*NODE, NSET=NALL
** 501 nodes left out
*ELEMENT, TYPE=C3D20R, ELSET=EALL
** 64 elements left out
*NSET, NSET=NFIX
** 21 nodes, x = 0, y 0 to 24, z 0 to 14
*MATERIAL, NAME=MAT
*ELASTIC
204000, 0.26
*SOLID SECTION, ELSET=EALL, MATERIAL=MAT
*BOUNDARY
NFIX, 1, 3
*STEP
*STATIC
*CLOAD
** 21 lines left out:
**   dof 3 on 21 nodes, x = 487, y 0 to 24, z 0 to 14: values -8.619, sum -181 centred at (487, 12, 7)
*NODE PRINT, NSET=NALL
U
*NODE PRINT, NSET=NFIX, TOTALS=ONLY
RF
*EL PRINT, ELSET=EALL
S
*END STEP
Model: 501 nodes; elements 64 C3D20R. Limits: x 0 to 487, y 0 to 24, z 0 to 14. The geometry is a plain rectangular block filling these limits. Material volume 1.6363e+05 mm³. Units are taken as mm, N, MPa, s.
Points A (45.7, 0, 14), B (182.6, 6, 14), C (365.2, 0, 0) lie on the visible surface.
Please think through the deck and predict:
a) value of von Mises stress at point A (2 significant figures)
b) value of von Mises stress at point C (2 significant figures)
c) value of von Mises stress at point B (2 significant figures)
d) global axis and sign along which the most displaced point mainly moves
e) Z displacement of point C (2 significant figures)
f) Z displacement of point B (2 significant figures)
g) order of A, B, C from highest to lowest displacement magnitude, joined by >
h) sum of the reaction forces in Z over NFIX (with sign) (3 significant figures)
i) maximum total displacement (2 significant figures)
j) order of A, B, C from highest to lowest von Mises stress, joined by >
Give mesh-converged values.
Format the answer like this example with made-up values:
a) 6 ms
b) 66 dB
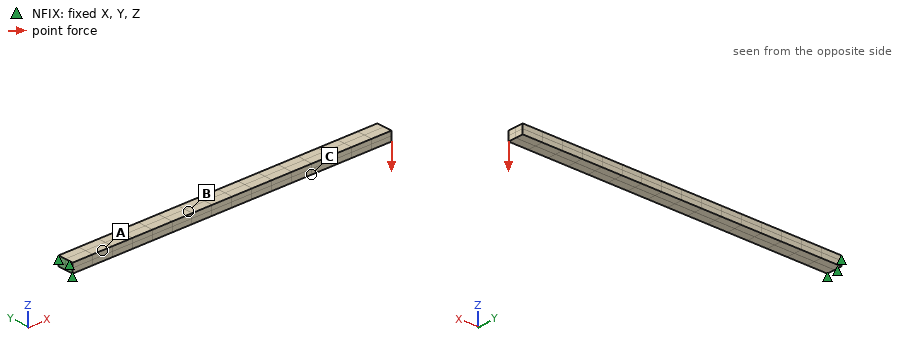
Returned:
a) 100 MPa
b) 28 MPa
c) 70 MPa
d) -Z
e) -3.9 mm
f) -1.1 mm
g) C > B > A
h) 181 N
i) 6.2 mm
j) A > B > C
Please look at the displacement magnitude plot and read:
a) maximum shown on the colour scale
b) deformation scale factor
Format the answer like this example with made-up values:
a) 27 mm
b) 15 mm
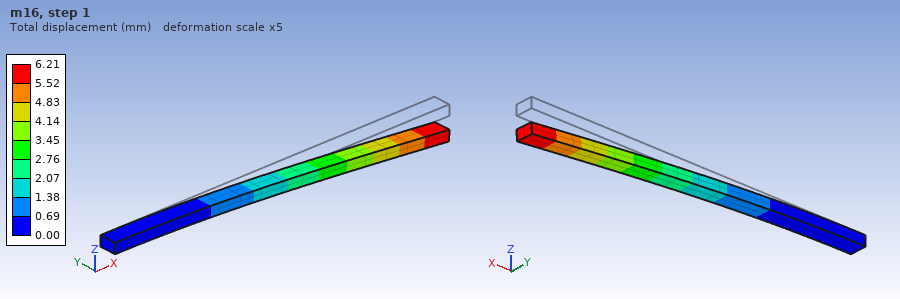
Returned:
a) 6.21 mm
b) 5
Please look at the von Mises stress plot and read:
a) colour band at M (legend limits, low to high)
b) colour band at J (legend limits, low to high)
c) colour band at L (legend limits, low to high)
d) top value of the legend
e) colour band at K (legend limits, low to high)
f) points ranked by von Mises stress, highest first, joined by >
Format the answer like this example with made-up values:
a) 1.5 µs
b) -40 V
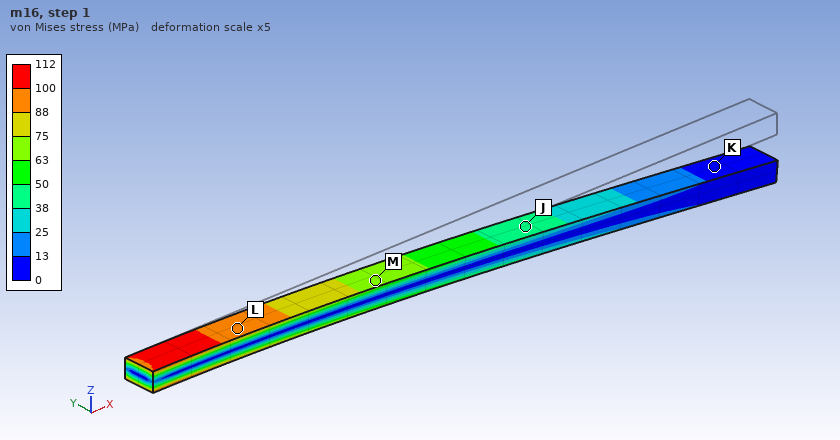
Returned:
a) 63 to 75 MPa
b) 38 to 50 MPa
c) 88 to 100 MPa
d) 112 MPa
e) 0 to 13 MPa
f) L > M > J > K
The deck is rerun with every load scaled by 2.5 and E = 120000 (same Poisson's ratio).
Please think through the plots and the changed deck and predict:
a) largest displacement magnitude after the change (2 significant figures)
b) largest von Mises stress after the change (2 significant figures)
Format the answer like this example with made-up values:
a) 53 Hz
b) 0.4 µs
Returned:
a) 26 mm
b) 280 MPa
